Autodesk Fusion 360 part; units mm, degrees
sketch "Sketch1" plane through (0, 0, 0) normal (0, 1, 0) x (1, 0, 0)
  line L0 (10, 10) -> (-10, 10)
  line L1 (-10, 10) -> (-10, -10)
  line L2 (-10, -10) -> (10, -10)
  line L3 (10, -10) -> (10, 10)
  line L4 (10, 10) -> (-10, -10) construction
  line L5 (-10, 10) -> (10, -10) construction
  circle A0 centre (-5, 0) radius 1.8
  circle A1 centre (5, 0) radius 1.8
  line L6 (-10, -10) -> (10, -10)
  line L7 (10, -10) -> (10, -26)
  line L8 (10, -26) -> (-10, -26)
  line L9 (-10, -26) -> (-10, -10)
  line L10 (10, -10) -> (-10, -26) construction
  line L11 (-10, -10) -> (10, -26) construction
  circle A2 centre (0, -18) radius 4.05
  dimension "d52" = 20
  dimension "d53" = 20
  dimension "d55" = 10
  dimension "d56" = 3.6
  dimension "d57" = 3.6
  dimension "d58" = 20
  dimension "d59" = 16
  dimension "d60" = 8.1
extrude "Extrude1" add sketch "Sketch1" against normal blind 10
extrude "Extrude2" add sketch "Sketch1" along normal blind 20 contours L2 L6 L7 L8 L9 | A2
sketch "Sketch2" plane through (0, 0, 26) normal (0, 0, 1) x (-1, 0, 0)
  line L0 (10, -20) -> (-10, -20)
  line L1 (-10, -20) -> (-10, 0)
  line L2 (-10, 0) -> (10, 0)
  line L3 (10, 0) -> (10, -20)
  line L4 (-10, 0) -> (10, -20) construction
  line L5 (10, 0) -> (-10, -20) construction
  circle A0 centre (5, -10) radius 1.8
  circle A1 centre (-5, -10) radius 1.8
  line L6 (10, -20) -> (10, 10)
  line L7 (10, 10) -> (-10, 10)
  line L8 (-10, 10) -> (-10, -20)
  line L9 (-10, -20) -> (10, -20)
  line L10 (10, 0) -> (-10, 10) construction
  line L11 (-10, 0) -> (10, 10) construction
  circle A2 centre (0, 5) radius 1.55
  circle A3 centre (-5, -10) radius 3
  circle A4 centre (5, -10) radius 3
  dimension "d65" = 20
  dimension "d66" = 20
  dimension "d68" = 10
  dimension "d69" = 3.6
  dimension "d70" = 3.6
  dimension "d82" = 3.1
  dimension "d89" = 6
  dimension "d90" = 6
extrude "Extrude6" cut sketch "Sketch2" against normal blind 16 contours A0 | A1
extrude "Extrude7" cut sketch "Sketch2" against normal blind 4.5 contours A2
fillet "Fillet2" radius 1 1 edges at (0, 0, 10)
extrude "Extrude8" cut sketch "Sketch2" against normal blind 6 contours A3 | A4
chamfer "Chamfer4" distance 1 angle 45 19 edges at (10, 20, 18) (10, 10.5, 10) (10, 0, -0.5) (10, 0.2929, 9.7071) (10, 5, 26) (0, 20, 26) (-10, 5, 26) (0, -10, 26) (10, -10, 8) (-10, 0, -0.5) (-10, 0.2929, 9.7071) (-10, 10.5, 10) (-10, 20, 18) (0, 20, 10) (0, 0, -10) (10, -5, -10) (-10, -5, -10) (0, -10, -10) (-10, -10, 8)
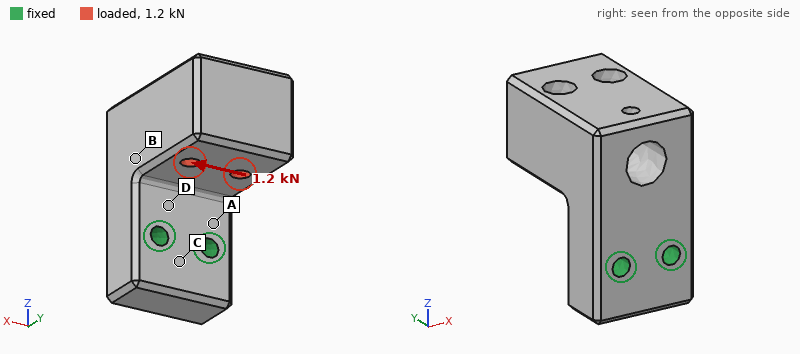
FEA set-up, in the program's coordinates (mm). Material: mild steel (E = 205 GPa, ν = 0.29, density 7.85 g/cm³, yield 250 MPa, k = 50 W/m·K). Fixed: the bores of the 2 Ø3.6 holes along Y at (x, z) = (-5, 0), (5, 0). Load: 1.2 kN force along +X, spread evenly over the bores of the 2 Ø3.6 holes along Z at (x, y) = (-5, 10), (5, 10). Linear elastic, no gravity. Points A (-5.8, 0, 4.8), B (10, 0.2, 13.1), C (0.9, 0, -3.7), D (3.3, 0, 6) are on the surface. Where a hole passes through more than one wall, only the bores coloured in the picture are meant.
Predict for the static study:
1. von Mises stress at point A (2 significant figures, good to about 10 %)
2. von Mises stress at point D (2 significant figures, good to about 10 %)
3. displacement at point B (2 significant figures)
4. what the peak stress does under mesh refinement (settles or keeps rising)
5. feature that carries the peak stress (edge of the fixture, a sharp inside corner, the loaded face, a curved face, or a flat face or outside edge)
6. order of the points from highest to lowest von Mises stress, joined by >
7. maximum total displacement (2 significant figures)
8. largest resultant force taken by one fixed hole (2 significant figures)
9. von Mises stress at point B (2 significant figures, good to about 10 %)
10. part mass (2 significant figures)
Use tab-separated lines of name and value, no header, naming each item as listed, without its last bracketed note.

von Mises stress at point A	45 MPa
von Mises stress at point D	55 MPa
displacement at point B	6.4 µm
what the peak stress does under mesh refinement	keeps rising
feature that carries the peak stress	edge of the fixture
order of the points from highest to lowest von Mises stress, joined by >	D > A > B > C
maximum total displacement	16 µm
largest resultant force taken by one fixed hole	1.8 kN
von Mises stress at point B	18 MPa
part mass	95 g
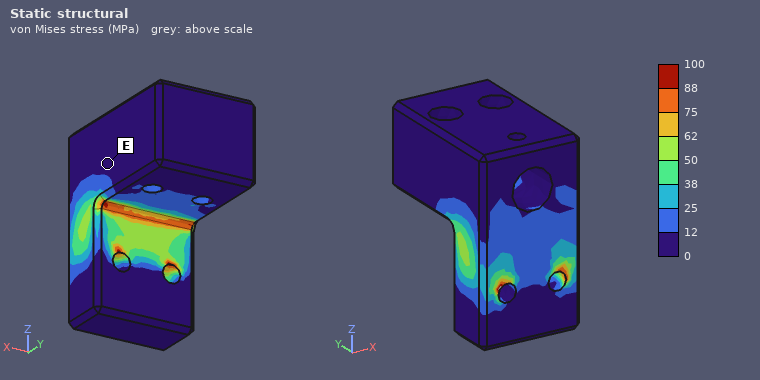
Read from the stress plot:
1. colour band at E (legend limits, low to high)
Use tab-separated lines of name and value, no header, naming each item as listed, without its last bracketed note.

colour band at E	0 to 12 MPa
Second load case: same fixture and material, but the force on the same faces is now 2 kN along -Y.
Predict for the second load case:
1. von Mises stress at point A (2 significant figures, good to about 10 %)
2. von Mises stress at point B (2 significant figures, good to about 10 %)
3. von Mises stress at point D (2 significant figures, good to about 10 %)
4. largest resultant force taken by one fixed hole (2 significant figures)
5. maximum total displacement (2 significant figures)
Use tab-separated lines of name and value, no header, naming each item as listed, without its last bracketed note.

von Mises stress at point A	69 MPa
von Mises stress at point B	17 MPa
von Mises stress at point D	55 MPa
largest resultant force taken by one fixed hole	1.0 kN
maximum total displacement	23 µm
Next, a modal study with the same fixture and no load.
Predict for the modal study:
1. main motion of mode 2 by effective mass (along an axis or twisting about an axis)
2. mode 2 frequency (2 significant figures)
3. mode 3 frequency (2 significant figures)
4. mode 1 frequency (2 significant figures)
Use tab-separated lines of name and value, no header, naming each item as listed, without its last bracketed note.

main motion of mode 2 by effective mass	along X
mode 2 frequency	7100 Hz
mode 3 frequency	14 kHz
mode 1 frequency	5100 Hz
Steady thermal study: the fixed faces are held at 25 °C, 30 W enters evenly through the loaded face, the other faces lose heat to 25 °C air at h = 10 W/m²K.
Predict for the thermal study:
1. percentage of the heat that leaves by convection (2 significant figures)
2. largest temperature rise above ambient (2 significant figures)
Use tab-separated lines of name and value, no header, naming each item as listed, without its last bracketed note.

percentage of the heat that leaves by convection	5.5 %
largest temperature rise above ambient	73 K
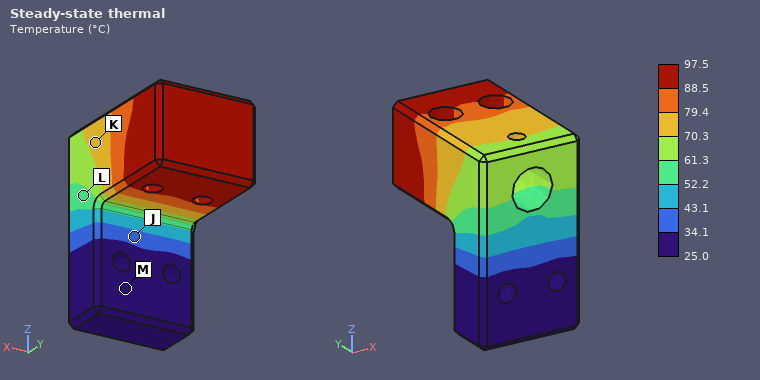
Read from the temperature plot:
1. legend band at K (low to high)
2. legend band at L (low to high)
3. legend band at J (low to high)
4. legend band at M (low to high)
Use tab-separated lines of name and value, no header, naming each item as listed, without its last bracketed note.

legend band at K	70.3 to 79.4 °C
legend band at L	52.2 to 61.3 °C
legend band at J	34.1 to 43.1 °C
legend band at M	25.0 to 34.1 °C
